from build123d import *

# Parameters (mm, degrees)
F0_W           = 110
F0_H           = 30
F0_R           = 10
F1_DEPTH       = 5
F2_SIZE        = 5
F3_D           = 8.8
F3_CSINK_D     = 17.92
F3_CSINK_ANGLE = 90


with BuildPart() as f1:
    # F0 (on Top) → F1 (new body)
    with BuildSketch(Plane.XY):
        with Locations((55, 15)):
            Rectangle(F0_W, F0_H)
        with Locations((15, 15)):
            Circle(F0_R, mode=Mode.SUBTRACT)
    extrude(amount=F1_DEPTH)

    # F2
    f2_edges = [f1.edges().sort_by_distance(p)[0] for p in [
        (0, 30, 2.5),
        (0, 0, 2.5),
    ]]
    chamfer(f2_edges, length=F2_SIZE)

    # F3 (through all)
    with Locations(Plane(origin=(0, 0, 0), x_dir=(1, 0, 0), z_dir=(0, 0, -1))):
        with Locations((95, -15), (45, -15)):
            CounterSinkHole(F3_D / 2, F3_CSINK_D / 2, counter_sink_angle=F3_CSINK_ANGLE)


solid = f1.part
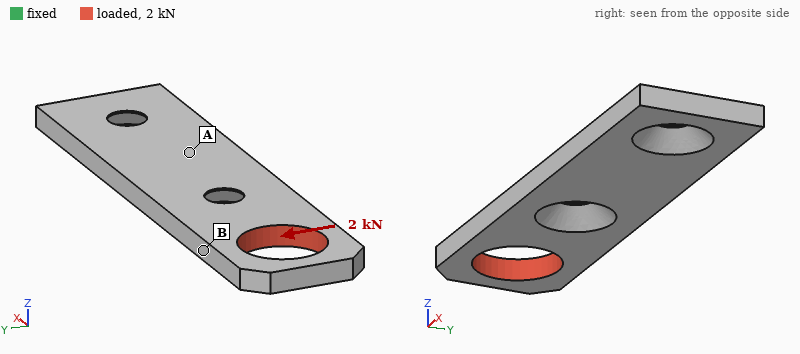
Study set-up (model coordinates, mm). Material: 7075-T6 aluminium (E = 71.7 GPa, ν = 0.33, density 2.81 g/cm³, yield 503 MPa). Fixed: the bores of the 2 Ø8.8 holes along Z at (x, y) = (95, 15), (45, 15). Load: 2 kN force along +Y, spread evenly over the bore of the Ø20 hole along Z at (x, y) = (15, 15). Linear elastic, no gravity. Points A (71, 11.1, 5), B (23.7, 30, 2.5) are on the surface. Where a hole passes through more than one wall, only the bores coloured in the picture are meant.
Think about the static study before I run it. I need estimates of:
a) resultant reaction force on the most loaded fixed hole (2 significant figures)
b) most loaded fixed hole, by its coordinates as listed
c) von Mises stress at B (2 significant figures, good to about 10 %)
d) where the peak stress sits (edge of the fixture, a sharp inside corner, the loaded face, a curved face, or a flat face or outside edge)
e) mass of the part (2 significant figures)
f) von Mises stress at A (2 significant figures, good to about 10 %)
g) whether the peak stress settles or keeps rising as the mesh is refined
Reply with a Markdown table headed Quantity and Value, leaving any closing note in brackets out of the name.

| Quantity | Value |
|---|---|
| resultant reaction force on the most loaded fixed hole | 2.9 kN |
| most loaded fixed hole, by its coordinates as listed | (45, 15) |
| von Mises stress at B | 99 MPa |
| where the peak stress sits | edge of the fixture |
| mass of the part | 38 g |
| von Mises stress at A | 35 MPa |
| whether the peak stress settles or keeps rising as the mesh is refined | keeps rising |
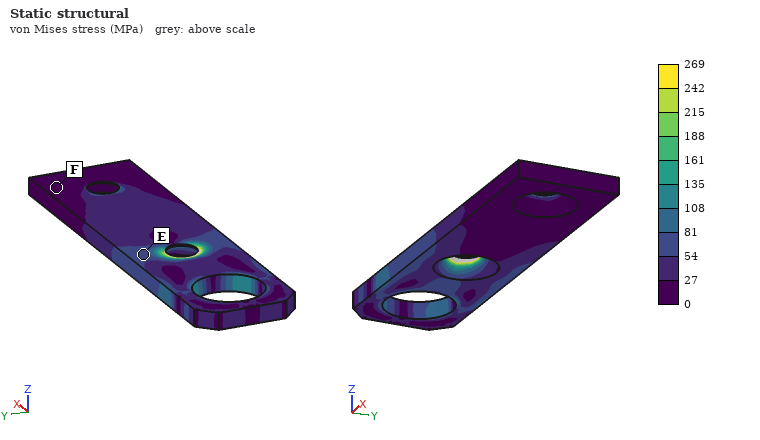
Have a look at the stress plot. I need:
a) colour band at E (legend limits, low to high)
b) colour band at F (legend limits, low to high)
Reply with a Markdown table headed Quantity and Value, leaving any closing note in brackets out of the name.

| Quantity | Value |
|---|---|
| colour band at E | 54 to 81 MPa |
| colour band at F | 0 to 27 MPa |
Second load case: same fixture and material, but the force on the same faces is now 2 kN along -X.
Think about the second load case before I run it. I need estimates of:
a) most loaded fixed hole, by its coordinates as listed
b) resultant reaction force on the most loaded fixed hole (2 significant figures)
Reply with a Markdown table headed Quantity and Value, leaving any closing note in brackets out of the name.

| Quantity | Value |
|---|---|
| most loaded fixed hole, by its coordinates as listed | (45, 15) |
| resultant reaction force on the most loaded fixed hole | 1.3 kN |
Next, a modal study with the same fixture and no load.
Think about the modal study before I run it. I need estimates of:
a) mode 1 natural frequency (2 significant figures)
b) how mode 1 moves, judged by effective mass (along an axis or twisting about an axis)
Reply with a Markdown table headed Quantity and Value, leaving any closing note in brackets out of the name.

| Quantity | Value |
|---|---|
| mode 1 natural frequency | 1800 Hz |
| how mode 1 moves, judged by effective mass | along Z |
